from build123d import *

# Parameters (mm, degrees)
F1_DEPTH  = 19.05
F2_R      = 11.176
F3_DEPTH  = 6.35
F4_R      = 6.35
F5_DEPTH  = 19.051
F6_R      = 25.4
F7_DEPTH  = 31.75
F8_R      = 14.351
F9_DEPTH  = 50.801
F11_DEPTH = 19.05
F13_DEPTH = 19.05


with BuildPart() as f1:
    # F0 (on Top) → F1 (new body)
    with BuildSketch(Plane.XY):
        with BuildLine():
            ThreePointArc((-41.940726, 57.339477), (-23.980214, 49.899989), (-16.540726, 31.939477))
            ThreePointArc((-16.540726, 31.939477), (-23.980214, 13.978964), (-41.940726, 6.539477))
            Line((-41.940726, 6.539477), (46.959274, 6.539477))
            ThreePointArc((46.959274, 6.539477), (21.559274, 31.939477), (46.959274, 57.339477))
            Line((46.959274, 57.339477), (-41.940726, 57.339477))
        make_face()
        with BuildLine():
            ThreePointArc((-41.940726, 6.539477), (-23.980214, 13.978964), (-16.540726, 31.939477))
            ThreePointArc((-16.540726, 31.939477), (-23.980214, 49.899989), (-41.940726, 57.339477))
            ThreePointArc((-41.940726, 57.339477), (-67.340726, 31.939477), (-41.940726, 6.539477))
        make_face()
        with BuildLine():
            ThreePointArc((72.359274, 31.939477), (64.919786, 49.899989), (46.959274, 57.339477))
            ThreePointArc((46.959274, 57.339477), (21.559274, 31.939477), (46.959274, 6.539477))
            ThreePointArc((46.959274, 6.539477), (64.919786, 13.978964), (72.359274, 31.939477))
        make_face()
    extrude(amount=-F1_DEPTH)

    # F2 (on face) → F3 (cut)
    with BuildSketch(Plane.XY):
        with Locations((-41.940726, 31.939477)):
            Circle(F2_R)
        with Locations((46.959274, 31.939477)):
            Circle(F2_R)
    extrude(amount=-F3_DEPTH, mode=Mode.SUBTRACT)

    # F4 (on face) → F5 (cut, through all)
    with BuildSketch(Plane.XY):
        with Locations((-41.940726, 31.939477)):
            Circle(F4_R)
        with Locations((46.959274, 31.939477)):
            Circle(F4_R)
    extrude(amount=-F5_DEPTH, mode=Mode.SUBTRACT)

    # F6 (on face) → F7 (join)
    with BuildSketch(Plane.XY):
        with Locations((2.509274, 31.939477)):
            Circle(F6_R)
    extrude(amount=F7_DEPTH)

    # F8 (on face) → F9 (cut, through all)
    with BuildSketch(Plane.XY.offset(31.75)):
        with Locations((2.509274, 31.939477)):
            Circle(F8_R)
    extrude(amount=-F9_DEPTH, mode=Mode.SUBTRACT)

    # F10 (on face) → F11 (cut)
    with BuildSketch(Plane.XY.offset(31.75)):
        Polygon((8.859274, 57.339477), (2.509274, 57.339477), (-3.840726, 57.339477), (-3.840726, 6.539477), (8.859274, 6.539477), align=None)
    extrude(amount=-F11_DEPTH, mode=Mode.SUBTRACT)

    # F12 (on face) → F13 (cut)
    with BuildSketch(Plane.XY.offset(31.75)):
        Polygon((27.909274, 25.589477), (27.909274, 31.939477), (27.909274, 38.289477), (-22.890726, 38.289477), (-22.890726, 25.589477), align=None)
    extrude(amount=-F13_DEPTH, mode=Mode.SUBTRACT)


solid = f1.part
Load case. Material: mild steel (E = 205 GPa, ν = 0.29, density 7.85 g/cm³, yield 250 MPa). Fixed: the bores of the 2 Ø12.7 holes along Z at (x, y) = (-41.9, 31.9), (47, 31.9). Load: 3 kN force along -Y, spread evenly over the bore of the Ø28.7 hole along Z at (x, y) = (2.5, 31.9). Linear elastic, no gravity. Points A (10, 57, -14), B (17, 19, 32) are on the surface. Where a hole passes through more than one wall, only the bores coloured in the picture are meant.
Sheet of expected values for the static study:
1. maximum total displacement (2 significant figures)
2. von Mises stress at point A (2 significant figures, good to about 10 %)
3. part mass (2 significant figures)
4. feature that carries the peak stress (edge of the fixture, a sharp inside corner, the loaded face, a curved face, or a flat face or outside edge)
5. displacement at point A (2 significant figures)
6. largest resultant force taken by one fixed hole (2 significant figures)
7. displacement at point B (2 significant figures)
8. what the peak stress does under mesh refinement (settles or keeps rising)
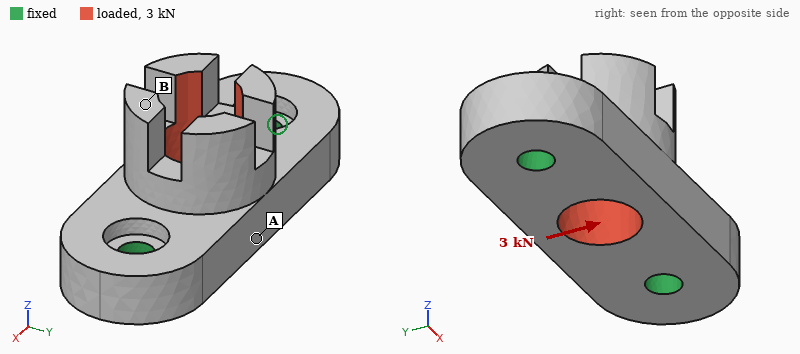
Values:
8.0 µm
6.0 MPa
1.1 kg
edge of the fixture
2.9 µm
1.5 kN
7.2 µm
keeps rising
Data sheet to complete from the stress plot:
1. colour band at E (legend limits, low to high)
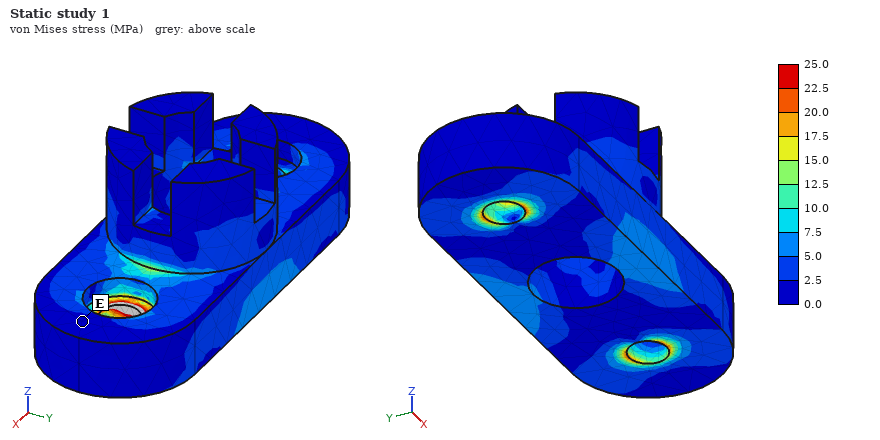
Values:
0.0 to 2.5 MPa
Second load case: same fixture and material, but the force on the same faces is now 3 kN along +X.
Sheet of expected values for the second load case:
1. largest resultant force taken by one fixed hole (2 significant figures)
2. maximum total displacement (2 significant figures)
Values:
1.6 kN
2.5 µm
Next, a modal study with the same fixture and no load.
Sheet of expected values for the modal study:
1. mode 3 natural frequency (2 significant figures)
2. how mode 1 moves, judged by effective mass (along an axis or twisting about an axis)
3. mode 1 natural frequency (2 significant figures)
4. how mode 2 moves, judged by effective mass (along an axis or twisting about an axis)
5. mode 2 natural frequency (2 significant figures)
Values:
8500 Hz
along Y
4800 Hz
along Z
7500 Hz
